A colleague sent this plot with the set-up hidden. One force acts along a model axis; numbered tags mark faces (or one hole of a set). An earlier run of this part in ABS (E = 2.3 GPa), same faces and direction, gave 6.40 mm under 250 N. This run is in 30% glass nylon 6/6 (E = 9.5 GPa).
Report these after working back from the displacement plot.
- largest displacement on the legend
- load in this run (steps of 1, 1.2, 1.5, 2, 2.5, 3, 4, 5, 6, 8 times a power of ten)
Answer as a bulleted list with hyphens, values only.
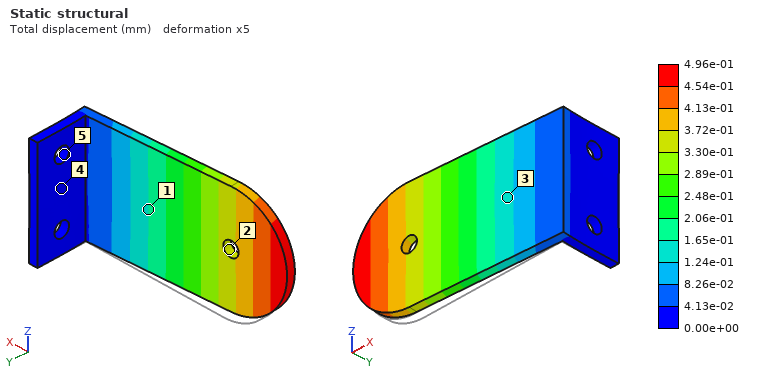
- 4.96e-01 mm
- 80 N
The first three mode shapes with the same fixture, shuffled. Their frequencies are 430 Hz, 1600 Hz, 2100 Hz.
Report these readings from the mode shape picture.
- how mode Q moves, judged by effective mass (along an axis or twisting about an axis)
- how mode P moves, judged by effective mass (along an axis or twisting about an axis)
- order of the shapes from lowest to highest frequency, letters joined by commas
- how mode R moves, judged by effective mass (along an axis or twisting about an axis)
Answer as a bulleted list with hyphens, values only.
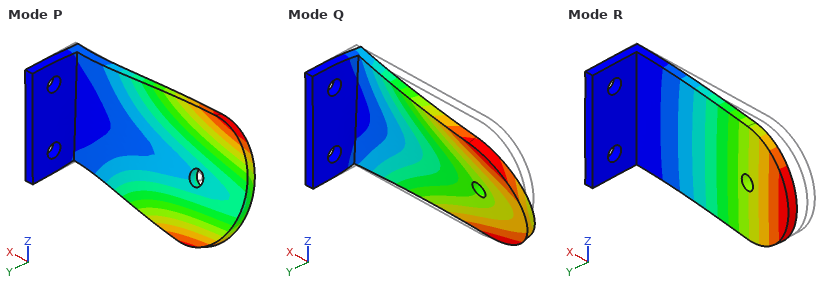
- along Z
- along Z
- R, Q, P
- along Y
